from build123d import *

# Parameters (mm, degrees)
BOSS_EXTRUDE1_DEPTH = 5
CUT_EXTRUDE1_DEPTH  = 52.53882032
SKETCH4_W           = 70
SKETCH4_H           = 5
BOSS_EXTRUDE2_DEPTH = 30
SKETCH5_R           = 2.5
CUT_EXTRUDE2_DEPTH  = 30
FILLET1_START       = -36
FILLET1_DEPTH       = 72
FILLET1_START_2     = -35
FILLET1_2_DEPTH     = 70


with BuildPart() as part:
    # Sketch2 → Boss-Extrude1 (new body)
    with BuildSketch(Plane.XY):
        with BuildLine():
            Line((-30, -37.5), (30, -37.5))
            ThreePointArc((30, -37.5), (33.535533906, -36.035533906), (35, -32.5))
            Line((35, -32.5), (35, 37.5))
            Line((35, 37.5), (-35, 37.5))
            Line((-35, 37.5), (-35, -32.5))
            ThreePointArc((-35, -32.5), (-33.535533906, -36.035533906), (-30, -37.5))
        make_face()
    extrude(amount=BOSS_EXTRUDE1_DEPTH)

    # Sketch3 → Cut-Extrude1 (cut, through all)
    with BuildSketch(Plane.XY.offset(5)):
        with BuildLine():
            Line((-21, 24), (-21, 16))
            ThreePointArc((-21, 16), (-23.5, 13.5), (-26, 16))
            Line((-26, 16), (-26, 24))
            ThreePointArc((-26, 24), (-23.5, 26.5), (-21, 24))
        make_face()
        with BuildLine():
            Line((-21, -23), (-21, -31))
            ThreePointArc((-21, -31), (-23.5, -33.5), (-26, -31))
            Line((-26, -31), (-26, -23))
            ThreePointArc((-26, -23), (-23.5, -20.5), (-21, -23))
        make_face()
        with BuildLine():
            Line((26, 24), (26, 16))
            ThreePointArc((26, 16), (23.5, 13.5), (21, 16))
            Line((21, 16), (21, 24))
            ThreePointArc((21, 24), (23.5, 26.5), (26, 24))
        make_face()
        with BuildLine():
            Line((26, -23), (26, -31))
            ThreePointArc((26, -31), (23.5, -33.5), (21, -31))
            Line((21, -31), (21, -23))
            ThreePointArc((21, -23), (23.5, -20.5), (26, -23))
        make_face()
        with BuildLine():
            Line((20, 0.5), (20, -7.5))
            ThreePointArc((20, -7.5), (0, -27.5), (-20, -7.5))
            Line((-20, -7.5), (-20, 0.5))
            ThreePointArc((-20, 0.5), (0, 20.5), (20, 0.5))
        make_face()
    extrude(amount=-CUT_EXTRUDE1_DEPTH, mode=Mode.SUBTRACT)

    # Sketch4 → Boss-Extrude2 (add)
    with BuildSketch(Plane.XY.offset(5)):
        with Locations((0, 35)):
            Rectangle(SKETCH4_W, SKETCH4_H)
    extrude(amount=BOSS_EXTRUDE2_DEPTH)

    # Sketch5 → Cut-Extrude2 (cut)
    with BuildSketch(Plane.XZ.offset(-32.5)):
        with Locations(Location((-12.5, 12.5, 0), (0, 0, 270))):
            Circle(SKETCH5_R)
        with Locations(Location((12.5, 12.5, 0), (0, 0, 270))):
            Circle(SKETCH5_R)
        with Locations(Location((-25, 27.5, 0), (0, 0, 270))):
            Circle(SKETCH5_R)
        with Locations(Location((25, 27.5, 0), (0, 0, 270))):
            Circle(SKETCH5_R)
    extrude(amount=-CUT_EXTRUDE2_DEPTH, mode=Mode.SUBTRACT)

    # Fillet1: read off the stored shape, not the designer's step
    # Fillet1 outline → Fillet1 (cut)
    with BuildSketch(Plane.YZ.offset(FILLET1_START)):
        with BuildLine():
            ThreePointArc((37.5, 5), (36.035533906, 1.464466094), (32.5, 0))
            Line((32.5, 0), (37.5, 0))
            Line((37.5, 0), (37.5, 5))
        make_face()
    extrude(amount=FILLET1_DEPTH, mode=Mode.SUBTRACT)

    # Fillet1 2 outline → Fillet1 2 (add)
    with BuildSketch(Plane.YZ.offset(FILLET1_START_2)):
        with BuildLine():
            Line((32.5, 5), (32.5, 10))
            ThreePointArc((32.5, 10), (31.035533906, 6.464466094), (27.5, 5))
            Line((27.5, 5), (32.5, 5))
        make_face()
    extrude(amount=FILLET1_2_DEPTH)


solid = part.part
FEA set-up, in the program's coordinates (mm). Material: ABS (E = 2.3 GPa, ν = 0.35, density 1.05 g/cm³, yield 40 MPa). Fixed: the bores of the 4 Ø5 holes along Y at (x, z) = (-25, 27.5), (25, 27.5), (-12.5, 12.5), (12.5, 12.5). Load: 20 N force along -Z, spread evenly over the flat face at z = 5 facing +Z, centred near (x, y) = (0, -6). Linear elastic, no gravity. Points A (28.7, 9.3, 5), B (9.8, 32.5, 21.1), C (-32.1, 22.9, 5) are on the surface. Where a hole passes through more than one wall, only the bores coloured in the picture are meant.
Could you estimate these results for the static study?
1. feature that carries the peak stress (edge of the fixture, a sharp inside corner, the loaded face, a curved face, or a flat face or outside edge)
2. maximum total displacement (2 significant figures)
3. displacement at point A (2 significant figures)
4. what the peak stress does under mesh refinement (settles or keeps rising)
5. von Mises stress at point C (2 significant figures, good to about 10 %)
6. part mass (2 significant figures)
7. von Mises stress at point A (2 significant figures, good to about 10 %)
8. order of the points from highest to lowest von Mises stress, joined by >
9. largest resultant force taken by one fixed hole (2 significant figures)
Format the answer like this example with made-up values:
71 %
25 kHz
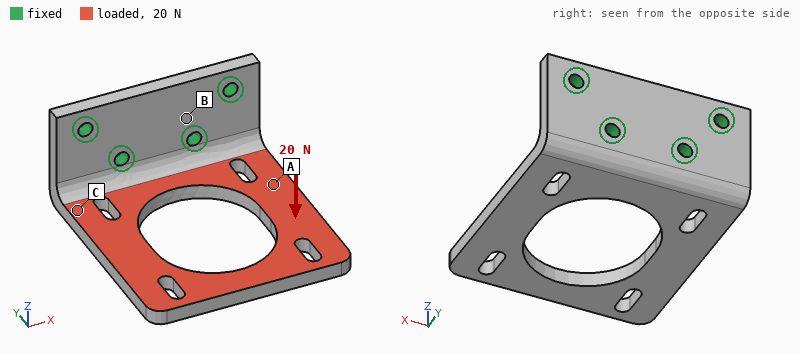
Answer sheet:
edge of the fixture
1.3 mm
0.24 mm
keeps rising
3.4 MPa
29 g
2.7 MPa
C > A > B
13 N
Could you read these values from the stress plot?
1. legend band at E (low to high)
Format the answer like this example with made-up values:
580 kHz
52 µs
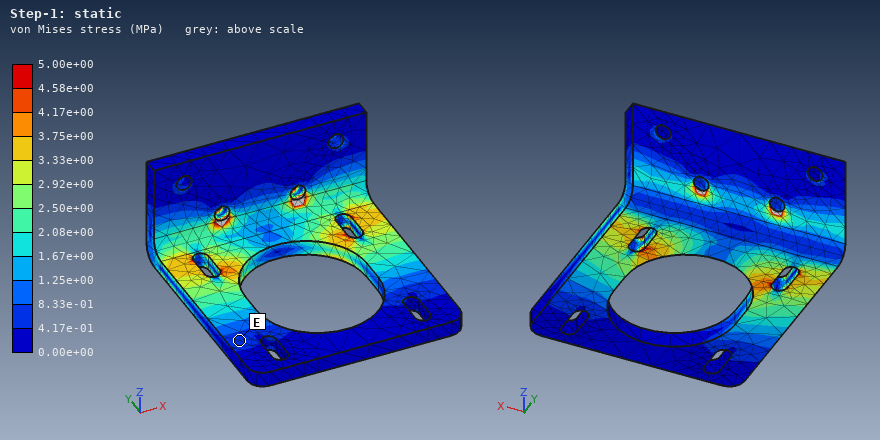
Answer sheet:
4.17e-01 to 8.33e-01 MPa
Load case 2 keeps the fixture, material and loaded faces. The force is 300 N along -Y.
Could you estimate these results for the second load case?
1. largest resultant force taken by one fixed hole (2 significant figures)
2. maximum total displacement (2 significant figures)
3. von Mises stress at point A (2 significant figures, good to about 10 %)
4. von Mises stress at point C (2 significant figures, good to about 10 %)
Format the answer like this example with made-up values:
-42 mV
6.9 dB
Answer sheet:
160 N
0.98 mm
4.5 MPa
4.5 MPa
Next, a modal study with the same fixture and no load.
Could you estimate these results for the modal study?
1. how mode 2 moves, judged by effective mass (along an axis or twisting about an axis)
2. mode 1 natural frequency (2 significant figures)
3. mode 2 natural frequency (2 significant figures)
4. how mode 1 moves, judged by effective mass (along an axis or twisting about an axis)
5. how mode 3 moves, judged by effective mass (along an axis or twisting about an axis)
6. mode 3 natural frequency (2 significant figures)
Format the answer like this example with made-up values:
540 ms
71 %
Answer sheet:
twisting about Y
200 Hz
420 Hz
along Z
along X
710 Hz
